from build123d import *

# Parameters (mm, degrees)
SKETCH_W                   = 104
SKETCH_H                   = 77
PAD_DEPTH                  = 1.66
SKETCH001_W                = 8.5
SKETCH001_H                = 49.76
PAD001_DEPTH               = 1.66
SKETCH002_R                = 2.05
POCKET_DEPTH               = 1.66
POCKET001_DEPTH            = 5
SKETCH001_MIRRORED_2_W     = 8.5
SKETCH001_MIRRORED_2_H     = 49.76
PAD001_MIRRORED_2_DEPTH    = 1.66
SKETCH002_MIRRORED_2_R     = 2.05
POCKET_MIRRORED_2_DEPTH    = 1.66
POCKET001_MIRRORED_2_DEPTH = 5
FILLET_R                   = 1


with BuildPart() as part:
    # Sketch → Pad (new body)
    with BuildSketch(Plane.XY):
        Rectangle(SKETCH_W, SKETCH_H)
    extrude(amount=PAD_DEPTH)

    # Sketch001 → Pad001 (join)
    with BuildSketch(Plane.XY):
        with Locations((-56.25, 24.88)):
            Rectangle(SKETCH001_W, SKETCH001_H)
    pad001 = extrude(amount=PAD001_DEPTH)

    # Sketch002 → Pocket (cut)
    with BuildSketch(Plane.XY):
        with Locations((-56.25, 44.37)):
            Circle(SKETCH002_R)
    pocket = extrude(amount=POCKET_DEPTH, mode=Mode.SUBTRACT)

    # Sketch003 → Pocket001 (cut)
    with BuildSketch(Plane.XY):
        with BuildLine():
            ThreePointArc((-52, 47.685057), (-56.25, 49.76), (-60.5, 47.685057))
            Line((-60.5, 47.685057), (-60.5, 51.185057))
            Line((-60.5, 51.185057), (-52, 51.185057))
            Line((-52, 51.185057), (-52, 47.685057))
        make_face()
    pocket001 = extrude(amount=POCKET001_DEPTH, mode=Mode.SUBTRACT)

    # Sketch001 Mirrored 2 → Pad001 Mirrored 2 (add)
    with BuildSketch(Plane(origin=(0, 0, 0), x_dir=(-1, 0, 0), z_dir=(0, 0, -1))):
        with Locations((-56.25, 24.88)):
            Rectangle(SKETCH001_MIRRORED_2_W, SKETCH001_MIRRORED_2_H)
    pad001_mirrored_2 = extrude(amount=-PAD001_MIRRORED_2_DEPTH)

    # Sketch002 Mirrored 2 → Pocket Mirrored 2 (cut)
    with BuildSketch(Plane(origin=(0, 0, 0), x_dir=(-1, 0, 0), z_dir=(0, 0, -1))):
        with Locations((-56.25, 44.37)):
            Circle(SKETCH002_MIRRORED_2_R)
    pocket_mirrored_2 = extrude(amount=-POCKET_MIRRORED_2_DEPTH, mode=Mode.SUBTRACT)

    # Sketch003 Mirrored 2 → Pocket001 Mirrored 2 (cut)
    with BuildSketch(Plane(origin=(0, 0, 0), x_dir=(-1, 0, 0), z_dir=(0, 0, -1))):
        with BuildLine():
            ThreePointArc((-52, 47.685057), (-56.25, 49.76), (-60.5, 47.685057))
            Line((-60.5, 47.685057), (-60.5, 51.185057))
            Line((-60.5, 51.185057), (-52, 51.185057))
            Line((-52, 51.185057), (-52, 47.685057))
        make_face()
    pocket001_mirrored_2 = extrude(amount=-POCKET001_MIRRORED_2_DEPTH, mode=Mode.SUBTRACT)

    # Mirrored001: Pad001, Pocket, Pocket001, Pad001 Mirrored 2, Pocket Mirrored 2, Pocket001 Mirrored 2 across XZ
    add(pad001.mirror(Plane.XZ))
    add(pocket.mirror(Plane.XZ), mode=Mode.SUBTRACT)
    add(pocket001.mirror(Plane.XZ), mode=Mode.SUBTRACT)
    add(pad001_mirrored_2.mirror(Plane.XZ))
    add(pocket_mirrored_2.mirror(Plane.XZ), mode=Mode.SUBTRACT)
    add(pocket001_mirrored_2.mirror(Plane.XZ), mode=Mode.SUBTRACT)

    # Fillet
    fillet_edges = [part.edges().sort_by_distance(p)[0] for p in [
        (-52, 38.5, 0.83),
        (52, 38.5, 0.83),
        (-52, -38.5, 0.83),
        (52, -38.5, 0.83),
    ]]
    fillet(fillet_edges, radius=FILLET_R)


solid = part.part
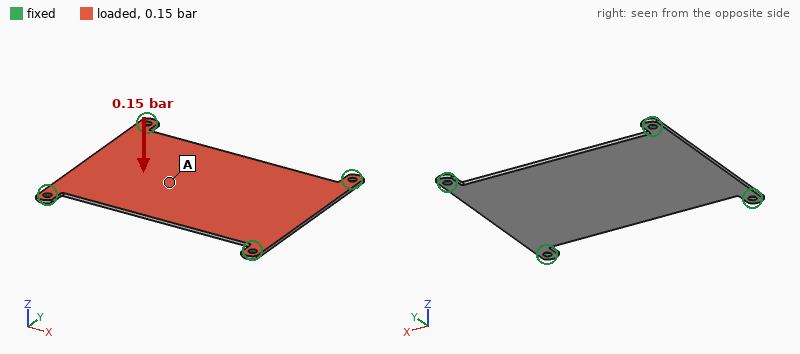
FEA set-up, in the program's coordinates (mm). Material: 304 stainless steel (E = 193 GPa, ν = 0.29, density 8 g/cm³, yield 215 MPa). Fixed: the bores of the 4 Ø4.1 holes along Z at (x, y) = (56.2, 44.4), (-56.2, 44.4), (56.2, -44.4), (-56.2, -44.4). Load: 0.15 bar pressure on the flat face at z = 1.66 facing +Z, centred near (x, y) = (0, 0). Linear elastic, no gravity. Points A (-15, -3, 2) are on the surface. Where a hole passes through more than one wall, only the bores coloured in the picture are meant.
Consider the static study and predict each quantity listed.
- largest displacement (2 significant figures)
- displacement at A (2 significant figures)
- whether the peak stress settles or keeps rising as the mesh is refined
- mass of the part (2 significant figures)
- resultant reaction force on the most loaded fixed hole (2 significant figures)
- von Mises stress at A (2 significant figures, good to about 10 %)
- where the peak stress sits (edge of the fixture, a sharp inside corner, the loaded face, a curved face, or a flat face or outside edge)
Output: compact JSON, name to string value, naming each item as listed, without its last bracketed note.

{"largest displacement": "0.23 mm", "displacement at A": "0.21 mm", "whether the peak stress settles or keeps rising as the mesh is refined": "keeps rising", "mass of the part": "130 g", "resultant reaction force on the most loaded fixed hole": "36 N", "von Mises stress at A": "21 MPa", "where the peak stress sits": "edge of the fixture"}
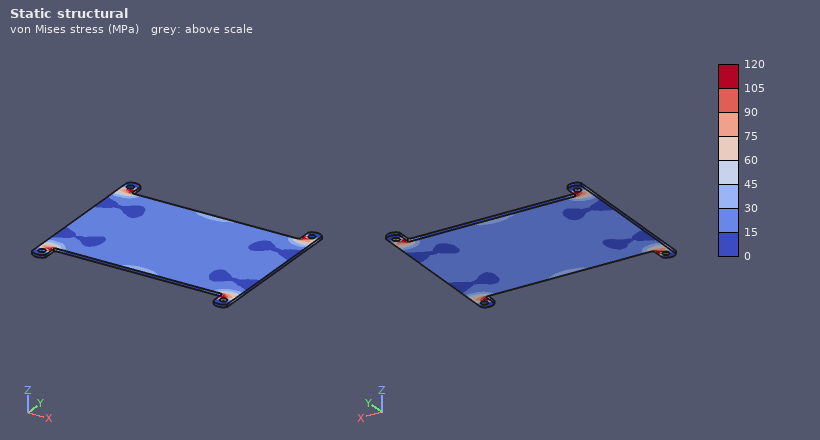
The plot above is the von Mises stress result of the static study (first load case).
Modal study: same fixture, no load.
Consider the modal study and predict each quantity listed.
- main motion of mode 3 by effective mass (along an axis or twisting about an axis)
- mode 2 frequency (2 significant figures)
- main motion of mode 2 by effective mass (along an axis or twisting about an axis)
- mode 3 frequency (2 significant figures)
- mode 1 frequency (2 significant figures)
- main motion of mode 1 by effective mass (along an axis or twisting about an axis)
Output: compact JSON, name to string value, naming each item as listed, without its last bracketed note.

{"main motion of mode 3 by effective mass": "twisting about Y", "mode 2 frequency": "820 Hz", "main motion of mode 2 by effective mass": "twisting about X", "mode 3 frequency": "950 Hz", "mode 1 frequency": "410 Hz", "main motion of mode 1 by effective mass": "along Z"}
